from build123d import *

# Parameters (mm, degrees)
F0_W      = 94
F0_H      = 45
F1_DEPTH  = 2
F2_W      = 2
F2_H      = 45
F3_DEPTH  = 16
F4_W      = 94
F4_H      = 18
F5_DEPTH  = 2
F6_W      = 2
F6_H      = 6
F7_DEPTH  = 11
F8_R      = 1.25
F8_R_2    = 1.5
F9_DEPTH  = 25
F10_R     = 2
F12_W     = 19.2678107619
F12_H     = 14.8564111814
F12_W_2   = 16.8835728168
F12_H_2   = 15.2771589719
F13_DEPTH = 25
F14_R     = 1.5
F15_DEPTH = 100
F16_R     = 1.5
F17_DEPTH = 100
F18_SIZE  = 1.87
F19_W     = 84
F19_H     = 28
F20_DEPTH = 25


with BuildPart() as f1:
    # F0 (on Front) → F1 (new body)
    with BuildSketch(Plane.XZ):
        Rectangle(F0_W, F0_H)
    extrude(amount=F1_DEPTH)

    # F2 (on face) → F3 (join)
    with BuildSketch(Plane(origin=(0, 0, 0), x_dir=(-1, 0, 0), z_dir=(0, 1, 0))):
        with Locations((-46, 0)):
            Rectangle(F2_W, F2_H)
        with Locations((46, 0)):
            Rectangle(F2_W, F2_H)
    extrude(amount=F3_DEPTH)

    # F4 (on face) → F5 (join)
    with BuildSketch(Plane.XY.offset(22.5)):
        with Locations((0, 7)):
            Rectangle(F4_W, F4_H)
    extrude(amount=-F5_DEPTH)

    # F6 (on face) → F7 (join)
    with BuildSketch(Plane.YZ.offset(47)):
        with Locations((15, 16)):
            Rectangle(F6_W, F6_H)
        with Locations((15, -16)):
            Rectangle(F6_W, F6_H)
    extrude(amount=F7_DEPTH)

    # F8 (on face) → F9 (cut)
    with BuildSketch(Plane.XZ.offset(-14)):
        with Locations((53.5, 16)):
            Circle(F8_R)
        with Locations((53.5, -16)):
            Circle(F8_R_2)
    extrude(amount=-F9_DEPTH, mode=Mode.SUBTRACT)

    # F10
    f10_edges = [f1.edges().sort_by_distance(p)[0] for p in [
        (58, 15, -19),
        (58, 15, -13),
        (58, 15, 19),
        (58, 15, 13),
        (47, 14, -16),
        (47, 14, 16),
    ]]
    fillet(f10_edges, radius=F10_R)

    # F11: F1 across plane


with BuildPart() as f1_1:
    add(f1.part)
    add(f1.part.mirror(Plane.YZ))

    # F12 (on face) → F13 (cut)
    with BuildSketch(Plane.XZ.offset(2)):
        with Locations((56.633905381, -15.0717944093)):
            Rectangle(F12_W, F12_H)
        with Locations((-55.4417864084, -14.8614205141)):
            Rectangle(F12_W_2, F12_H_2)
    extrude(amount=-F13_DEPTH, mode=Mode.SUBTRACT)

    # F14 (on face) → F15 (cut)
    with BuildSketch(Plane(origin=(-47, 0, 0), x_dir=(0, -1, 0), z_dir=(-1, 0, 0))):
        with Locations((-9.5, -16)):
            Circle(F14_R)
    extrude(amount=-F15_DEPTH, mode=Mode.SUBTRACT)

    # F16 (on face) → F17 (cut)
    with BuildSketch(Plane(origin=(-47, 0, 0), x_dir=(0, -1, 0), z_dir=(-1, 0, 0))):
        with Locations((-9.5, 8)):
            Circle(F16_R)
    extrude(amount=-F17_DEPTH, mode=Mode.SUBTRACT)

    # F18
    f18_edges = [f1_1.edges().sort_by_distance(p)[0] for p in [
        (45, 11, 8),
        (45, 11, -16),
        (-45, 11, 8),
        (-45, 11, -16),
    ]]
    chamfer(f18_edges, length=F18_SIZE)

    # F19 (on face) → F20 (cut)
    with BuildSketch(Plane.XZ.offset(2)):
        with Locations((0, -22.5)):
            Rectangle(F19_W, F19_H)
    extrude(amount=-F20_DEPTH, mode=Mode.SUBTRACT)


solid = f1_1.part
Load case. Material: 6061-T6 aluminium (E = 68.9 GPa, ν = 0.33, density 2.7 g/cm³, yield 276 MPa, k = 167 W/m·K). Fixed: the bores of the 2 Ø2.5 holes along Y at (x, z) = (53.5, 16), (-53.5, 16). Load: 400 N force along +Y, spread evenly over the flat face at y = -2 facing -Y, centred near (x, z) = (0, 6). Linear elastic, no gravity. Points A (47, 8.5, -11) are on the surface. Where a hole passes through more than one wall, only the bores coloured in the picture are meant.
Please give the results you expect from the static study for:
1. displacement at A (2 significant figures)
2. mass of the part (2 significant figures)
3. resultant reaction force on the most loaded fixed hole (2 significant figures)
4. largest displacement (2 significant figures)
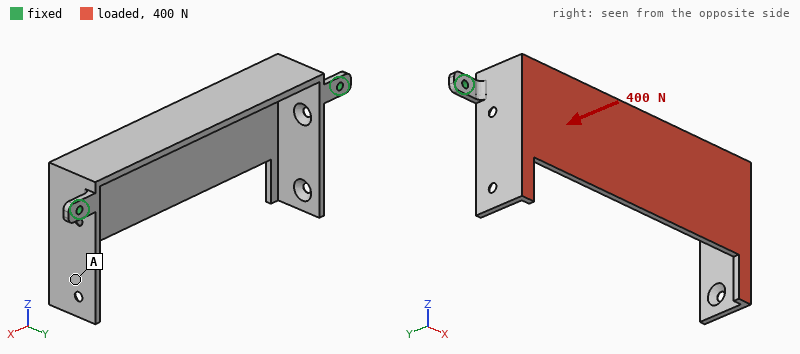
0.79 mm
32 g
240 N
1.2 mm
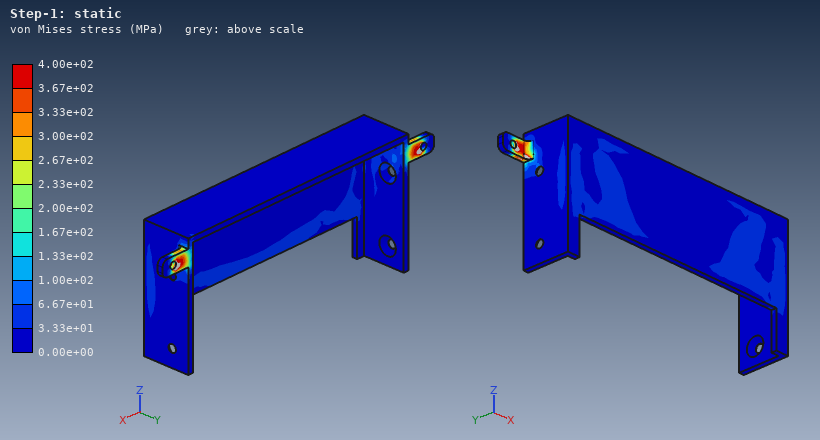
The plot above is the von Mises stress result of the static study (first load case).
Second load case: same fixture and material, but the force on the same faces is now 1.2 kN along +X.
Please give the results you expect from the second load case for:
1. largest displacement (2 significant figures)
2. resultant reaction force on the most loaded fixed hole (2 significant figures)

0.95 mm
650 N
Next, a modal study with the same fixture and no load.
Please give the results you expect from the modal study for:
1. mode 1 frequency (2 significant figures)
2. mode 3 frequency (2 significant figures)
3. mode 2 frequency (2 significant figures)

550 Hz
1700 Hz
980 Hz
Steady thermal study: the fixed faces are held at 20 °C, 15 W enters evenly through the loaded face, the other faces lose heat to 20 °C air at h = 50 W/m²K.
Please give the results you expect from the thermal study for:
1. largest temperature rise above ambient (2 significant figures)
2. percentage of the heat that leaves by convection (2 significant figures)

23 K
57 %
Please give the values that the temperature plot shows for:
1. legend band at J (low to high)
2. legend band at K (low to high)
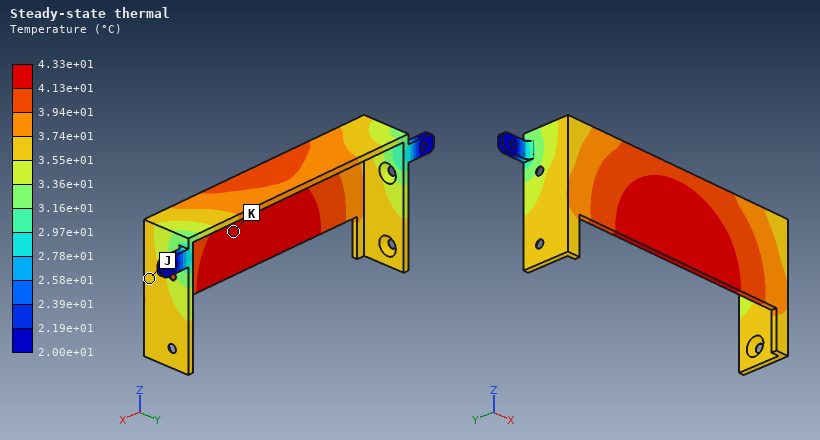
3.55e+01 to 3.74e+01 °C
4.13e+01 to 4.33e+01 °C
